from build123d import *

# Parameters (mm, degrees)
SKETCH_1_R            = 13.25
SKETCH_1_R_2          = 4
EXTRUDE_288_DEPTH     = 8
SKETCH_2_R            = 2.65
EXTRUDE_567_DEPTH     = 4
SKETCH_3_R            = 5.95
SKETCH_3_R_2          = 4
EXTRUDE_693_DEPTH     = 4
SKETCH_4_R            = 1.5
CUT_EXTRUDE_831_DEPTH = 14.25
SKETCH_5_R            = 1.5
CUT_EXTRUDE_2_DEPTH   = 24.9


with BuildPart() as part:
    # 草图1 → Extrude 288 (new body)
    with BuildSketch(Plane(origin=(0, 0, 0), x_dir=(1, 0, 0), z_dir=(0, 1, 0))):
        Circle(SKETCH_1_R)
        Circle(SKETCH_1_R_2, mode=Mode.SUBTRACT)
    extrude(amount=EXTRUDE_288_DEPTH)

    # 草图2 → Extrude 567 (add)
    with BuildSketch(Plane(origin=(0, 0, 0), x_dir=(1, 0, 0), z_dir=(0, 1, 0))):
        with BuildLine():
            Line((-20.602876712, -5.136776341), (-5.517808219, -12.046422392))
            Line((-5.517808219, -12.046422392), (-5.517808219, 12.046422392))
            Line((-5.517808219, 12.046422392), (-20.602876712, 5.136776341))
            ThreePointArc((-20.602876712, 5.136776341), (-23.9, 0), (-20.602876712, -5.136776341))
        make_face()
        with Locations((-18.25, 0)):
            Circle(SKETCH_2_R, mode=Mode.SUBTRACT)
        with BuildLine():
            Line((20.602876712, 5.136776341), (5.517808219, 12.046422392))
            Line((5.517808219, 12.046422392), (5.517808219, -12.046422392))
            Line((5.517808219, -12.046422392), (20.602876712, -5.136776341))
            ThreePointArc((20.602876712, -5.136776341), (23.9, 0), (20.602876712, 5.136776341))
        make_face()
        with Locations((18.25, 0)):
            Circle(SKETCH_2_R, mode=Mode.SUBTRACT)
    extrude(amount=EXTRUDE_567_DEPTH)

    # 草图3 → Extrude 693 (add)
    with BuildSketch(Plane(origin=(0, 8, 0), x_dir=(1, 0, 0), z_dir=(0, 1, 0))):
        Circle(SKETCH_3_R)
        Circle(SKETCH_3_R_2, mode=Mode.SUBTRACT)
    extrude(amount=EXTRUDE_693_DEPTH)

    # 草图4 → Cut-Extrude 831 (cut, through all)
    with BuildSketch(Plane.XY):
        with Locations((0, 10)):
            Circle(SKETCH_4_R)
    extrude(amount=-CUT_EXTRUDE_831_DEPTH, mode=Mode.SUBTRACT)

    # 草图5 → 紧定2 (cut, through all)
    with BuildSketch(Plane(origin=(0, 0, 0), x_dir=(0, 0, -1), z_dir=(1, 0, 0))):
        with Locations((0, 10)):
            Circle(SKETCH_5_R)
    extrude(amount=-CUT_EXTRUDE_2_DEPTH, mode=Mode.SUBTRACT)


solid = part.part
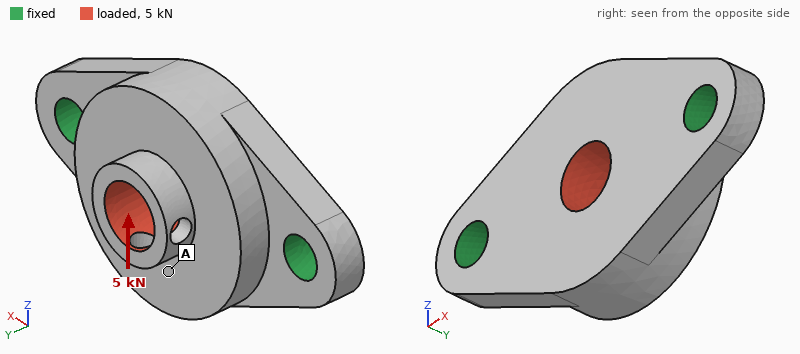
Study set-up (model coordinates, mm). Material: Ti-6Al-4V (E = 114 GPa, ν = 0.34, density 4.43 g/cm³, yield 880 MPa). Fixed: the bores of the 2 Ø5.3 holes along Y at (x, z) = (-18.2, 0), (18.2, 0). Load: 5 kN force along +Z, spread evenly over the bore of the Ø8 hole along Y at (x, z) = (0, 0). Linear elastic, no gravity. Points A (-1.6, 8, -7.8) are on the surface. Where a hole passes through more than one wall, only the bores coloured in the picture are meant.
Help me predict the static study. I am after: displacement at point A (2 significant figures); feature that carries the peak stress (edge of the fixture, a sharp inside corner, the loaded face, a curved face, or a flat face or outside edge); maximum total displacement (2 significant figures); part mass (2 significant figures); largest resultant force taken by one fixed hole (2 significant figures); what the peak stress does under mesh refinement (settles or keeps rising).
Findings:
42 µm
edge of the fixture
57 µm
23 g
2.5 kN
keeps rising
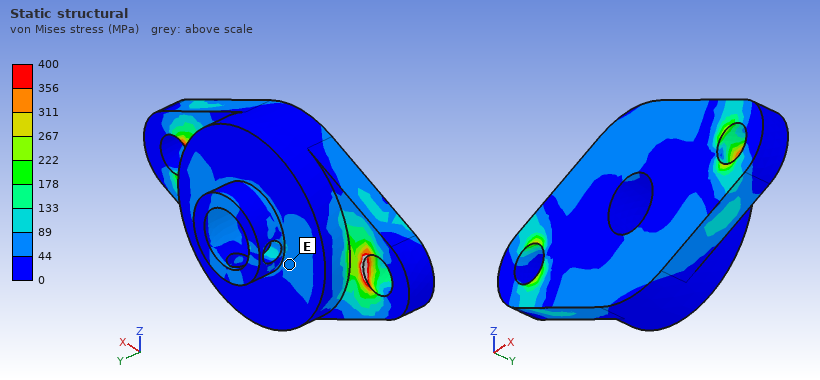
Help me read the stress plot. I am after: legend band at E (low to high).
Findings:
44 to 89 MPa
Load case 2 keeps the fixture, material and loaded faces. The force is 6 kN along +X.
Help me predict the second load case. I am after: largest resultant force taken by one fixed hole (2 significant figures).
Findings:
3.1 kN
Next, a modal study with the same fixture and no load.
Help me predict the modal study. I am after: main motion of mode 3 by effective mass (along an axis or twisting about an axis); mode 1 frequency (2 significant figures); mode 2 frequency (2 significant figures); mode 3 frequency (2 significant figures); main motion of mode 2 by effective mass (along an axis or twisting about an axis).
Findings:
along Z
11 kHz
16 kHz
28 kHz
along Y
